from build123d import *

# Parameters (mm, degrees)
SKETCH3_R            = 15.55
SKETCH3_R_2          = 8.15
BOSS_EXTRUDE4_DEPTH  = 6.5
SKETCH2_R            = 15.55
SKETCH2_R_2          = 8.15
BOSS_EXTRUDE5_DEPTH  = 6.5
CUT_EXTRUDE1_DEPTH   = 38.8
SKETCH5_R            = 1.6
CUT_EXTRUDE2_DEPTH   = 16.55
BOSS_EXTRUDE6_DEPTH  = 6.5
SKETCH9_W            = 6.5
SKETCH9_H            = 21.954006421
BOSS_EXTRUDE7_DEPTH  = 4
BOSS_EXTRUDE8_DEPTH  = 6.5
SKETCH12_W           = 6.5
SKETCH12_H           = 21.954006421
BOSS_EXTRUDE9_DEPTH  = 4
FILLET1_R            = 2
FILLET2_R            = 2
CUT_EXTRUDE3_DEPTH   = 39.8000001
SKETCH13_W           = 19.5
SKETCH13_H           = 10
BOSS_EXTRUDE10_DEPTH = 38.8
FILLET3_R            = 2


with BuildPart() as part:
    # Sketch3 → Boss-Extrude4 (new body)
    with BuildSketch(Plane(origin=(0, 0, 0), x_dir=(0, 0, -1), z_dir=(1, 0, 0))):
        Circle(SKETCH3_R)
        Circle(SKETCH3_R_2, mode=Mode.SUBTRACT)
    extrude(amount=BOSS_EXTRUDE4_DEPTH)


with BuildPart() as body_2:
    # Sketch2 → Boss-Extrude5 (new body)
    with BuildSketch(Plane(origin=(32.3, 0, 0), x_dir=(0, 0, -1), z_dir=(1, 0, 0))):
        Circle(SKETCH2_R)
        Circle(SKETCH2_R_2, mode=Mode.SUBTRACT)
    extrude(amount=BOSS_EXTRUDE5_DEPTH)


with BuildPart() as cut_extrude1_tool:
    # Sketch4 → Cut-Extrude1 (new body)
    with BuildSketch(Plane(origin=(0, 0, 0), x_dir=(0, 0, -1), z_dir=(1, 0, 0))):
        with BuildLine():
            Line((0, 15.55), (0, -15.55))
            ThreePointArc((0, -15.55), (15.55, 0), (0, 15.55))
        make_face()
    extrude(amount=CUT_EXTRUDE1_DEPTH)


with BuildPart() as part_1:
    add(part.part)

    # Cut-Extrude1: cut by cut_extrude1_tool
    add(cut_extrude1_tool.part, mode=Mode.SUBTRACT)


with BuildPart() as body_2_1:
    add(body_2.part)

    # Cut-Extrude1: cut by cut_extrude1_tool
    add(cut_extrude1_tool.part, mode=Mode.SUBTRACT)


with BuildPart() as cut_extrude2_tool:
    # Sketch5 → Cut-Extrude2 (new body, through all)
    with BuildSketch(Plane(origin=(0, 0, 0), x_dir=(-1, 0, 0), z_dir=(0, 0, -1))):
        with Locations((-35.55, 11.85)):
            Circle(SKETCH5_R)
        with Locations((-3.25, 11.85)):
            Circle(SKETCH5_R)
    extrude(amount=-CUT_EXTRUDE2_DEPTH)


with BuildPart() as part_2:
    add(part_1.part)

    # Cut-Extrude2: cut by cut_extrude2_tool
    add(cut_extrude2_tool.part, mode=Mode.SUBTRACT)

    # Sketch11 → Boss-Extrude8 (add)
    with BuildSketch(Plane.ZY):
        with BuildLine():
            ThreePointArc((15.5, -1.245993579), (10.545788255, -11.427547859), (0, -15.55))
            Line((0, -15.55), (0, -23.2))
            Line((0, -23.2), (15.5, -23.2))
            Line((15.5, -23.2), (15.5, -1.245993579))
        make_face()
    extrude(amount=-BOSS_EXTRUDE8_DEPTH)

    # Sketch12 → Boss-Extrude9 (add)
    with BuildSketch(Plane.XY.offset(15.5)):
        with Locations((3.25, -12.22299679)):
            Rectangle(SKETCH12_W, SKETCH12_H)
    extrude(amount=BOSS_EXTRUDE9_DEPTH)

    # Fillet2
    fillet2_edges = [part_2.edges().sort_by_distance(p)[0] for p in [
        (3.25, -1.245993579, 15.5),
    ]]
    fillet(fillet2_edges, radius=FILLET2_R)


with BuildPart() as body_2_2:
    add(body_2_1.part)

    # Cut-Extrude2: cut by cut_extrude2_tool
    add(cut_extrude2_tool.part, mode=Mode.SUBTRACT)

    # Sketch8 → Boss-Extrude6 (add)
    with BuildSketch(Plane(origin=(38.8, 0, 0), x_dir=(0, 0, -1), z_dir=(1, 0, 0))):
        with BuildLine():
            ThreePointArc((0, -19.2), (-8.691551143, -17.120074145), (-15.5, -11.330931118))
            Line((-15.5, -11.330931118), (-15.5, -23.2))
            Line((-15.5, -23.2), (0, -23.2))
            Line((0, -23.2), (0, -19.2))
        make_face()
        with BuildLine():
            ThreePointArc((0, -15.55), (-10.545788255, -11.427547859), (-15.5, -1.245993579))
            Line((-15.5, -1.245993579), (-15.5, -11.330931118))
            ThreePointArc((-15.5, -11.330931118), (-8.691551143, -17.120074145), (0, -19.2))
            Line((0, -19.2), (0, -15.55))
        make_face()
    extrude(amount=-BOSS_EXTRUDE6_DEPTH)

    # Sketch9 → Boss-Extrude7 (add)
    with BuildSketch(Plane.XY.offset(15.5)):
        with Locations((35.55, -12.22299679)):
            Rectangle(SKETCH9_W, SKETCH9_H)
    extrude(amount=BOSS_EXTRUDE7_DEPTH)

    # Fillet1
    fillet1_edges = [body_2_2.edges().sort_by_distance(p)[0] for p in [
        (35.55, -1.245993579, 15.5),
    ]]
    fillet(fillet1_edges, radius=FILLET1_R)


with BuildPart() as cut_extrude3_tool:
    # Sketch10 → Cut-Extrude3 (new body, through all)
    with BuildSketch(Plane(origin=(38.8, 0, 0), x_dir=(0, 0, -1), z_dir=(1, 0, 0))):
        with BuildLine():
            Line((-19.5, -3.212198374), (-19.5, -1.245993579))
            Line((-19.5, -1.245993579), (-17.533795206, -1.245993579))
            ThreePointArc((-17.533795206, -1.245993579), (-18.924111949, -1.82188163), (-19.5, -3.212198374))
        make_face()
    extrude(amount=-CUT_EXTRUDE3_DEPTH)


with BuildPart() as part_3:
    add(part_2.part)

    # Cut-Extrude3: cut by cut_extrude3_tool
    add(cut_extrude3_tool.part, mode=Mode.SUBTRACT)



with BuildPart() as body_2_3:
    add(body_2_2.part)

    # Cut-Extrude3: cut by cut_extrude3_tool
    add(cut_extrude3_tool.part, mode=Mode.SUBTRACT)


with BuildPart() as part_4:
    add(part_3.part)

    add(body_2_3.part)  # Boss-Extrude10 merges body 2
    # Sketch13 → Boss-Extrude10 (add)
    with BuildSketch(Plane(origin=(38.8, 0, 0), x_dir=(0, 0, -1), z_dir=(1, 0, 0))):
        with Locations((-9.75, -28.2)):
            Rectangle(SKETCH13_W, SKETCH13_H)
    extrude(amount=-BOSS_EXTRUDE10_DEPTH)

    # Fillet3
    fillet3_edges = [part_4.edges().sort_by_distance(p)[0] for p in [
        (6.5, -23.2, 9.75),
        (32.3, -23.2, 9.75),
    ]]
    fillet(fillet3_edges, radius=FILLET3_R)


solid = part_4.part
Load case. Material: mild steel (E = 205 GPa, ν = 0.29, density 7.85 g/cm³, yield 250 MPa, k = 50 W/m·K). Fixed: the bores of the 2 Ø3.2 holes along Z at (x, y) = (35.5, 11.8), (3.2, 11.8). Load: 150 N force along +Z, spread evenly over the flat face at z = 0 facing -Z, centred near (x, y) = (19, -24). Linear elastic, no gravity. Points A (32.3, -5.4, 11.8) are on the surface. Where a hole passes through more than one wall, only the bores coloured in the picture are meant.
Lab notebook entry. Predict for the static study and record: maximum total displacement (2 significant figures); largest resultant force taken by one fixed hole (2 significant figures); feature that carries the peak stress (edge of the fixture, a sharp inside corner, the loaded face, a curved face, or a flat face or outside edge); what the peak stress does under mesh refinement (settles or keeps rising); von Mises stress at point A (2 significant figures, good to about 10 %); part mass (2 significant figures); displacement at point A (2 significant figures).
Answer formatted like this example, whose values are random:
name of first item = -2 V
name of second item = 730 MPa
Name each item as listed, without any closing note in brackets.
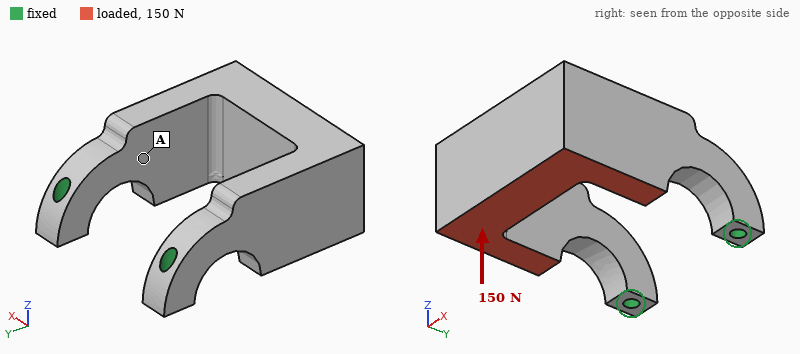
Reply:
maximum total displacement = 27 µm
largest resultant force taken by one fixed hole = 75 N
feature that carries the peak stress = edge of the fixture
what the peak stress does under mesh refinement = keeps rising
von Mises stress at point A = 7.3 MPa
part mass = 110 g
displacement at point A = 6.7 µm
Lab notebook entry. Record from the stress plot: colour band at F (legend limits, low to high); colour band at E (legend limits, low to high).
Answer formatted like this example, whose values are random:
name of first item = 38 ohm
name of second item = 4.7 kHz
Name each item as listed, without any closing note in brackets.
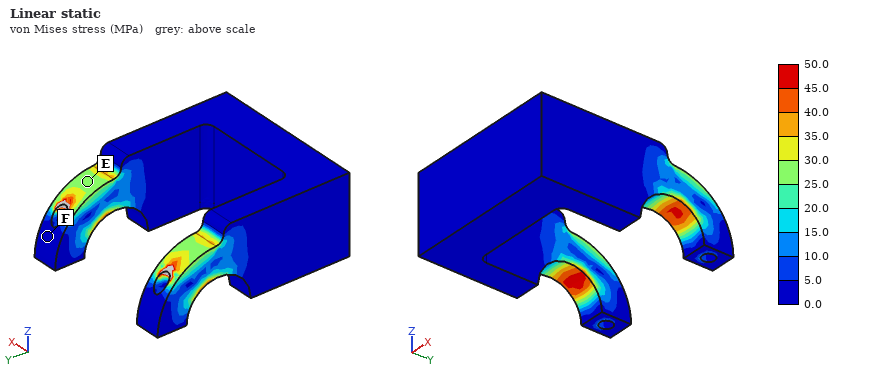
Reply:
colour band at F = 0.0 to 5.0 MPa
colour band at E = 25.0 to 30.0 MPa
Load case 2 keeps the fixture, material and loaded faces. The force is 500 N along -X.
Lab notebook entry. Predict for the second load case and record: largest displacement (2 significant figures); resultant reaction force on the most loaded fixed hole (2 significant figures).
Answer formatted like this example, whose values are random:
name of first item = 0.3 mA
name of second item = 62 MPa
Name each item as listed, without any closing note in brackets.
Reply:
largest displacement = 31 µm
resultant reaction force on the most loaded fixed hole = 440 N
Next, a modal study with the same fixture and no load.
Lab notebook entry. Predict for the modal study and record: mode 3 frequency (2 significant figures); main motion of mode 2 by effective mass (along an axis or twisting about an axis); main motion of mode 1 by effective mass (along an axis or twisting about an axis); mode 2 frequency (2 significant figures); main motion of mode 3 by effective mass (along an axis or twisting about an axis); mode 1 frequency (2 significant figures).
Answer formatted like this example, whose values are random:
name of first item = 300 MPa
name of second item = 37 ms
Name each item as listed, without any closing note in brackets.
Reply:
mode 3 frequency = 4600 Hz
main motion of mode 2 by effective mass = along X
main motion of mode 1 by effective mass = along Z
mode 2 frequency = 2500 Hz
main motion of mode 3 by effective mass = twisting about Y
mode 1 frequency = 1400 Hz
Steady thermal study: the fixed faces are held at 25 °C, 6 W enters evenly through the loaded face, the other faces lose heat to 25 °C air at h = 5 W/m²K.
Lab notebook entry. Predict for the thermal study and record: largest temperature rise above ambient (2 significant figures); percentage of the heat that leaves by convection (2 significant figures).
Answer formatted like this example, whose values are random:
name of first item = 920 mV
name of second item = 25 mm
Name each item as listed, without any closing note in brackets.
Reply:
largest temperature rise above ambient = 29 K
percentage of the heat that leaves by convection = 8.5 %
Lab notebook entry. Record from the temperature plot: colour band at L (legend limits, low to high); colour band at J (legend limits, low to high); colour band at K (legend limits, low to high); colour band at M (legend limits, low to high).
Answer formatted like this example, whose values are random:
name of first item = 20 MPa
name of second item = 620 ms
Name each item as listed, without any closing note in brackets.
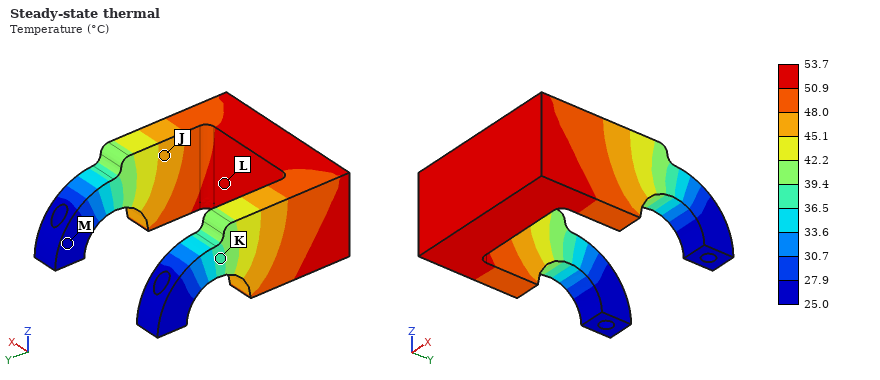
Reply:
colour band at L = 50.9 to 53.7 °C
colour band at J = 45.1 to 48.0 °C
colour band at K = 36.5 to 39.4 °C
colour band at M = 25.0 to 27.9 °C
